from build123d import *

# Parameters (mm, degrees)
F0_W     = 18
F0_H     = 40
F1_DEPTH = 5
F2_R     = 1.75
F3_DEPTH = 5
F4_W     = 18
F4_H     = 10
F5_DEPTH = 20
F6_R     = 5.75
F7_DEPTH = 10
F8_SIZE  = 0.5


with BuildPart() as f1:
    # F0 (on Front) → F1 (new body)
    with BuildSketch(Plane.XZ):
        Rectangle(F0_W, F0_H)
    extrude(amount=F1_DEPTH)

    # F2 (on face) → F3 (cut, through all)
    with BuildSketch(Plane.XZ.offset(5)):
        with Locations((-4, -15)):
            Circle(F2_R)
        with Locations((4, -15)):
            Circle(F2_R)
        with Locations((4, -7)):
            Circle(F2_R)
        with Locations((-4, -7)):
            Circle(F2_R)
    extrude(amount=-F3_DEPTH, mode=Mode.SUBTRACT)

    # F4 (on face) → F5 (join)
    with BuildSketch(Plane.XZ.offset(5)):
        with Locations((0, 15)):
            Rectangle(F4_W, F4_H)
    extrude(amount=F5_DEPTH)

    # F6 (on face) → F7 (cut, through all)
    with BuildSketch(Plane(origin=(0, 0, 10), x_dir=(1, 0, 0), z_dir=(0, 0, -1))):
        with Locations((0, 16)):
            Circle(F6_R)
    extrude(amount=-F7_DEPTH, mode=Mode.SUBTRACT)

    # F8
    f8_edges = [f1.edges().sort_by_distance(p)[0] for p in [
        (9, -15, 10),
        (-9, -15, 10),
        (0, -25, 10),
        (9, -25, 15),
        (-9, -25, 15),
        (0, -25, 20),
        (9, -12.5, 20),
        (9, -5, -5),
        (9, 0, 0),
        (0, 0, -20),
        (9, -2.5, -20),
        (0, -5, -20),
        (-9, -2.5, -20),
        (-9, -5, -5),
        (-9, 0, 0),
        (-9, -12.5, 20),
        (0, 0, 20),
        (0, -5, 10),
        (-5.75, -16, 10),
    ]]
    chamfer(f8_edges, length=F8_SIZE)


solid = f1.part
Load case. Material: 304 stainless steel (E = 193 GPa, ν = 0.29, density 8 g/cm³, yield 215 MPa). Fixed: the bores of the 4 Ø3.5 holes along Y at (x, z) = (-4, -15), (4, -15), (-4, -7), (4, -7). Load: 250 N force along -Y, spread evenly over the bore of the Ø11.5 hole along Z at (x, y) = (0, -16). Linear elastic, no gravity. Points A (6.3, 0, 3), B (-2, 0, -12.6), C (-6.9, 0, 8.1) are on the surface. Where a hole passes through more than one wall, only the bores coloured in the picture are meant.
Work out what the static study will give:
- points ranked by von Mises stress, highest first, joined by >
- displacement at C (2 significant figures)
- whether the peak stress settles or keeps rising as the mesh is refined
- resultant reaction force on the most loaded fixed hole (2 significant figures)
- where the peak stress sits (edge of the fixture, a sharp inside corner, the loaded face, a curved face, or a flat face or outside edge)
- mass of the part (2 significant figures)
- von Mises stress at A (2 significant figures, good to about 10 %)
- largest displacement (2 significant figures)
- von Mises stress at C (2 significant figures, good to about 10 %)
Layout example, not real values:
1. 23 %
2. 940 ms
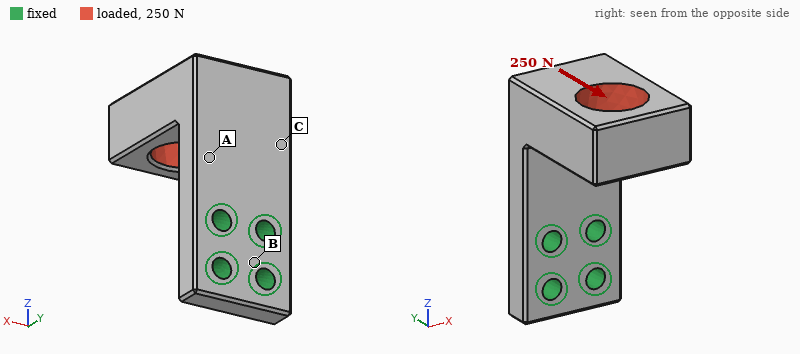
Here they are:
1. A > C > B
2. 13 µm
3. keeps rising
4. 160 N
5. edge of the fixture
6. 47 g
7. 41 MPa
8. 46 µm
9. 23 MPa
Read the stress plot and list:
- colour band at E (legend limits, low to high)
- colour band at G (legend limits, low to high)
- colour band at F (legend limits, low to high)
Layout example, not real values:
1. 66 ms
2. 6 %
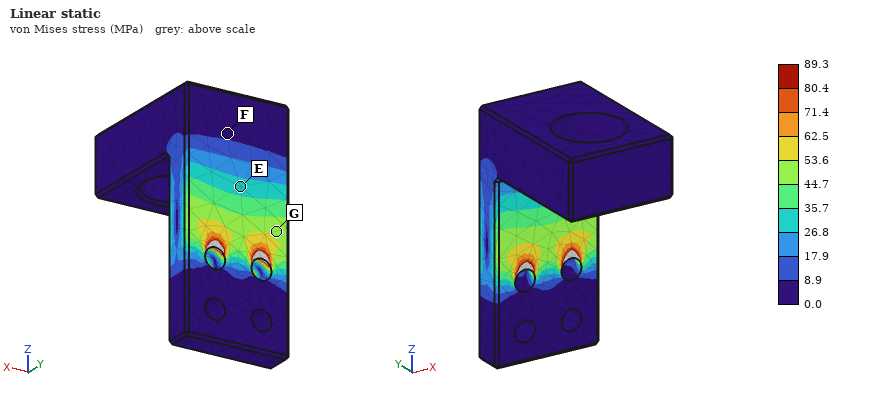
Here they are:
1. 26.8 to 35.7 MPa
2. 44.7 to 53.6 MPa
3. 0.0 to 8.9 MPa
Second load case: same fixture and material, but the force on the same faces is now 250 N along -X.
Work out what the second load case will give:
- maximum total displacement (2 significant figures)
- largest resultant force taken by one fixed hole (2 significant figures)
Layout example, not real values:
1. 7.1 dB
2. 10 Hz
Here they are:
1. 26 µm
2. 510 N
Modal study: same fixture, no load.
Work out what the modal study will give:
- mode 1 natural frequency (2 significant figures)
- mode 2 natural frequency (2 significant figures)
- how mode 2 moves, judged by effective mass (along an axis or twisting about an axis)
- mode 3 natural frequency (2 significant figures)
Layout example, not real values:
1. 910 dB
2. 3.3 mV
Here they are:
1. 2400 Hz
2. 4100 Hz
3. along X
4. 9100 Hz
